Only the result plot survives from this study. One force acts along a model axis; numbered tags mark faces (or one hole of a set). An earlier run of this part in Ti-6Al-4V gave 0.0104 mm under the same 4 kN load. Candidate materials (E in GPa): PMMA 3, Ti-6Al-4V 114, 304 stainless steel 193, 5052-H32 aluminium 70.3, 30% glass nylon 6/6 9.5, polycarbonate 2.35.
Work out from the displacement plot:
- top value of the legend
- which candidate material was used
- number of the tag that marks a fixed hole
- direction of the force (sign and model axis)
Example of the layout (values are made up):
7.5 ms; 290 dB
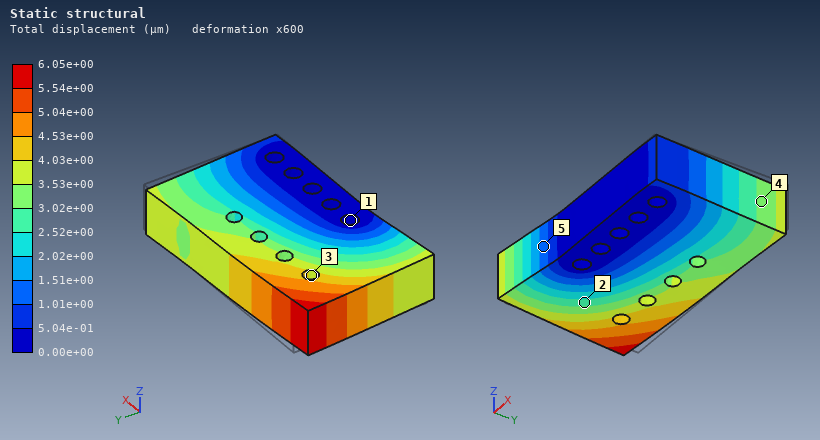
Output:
6.05e+00 µm; 304 stainless steel; 1; -X
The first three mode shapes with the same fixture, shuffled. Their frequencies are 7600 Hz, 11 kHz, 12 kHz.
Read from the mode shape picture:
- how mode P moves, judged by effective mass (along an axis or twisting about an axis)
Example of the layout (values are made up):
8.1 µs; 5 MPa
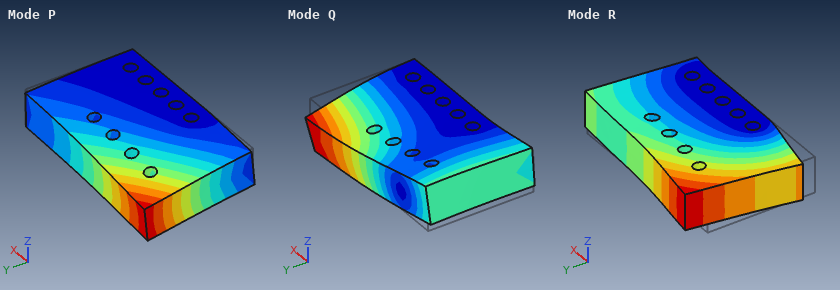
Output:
along Z
